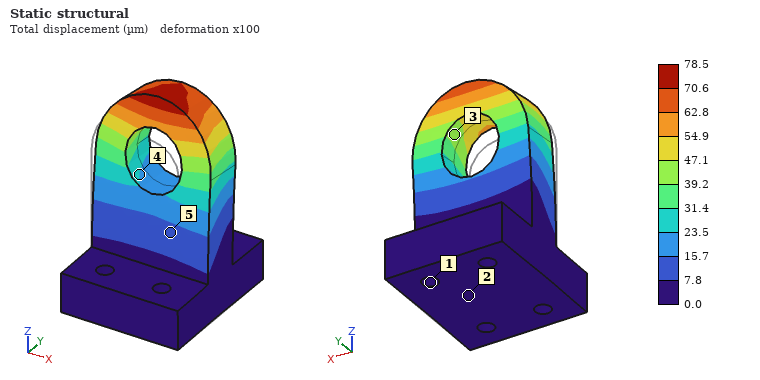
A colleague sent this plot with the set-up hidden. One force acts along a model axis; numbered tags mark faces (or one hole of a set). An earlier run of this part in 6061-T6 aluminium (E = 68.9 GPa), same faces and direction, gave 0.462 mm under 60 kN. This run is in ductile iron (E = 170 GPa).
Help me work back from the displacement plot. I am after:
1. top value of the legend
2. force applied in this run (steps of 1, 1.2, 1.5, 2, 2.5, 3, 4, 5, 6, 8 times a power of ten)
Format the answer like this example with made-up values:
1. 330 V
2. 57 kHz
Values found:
1. 78.5 µm
2. 25 kN
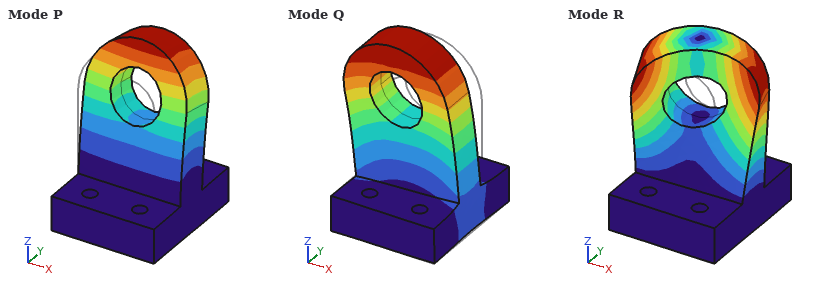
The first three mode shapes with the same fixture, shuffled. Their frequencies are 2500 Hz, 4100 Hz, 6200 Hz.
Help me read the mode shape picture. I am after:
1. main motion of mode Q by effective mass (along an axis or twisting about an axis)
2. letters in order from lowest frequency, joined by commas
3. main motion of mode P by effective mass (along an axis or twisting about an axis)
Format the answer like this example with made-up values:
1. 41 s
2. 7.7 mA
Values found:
1. along X
2. P, Q, R
3. along Y
